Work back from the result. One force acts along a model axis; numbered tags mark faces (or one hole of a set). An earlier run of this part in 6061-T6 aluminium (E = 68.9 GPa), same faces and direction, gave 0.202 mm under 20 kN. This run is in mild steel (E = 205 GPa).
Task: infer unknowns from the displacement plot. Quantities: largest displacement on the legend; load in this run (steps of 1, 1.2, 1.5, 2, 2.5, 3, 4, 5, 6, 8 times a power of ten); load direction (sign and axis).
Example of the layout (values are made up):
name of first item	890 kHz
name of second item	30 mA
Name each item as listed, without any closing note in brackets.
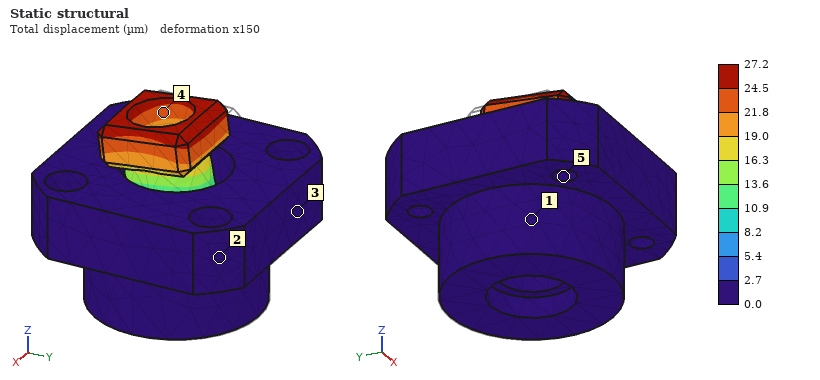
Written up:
largest displacement on the legend	27.2 µm
load in this run	8 kN
load direction	-Y
